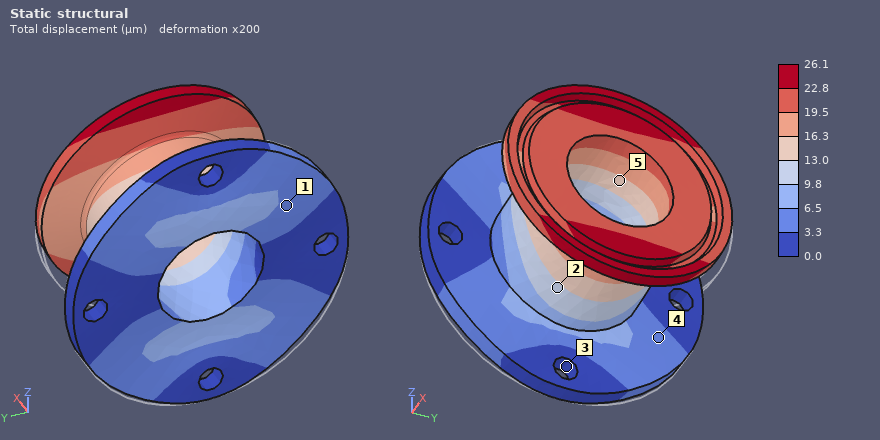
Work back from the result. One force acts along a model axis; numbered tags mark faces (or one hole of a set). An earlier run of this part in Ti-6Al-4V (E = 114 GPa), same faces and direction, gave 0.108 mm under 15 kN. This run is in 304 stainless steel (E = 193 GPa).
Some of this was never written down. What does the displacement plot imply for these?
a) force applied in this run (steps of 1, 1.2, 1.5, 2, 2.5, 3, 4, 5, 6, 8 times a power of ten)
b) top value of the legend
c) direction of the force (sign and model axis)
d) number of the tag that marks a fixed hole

6 kN
26.1 µm
+Z
3
